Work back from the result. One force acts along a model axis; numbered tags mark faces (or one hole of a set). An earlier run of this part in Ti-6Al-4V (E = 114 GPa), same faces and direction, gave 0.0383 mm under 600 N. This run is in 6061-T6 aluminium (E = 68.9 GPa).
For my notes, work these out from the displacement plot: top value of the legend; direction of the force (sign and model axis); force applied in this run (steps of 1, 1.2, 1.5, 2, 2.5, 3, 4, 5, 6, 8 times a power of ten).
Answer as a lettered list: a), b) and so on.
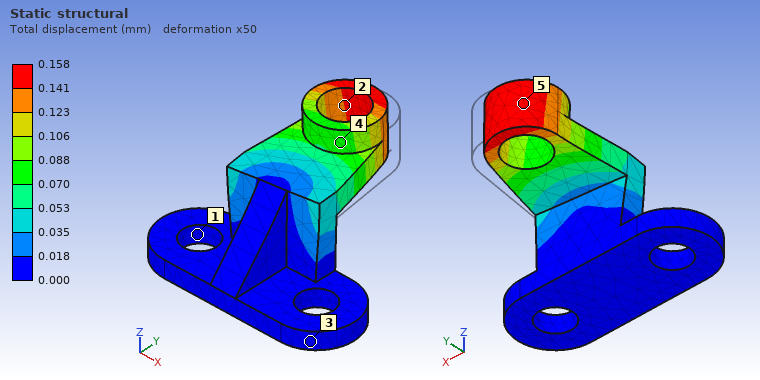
a) 0.158 mm
b) -X
c) 1.5 kN
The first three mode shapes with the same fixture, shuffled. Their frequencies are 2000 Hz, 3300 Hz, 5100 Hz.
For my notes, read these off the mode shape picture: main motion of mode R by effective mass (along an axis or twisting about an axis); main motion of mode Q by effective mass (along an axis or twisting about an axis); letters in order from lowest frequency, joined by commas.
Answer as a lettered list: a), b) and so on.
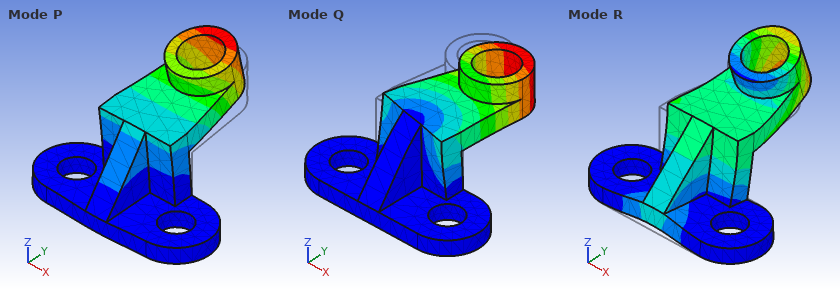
a) along Y
b) along X
c) P, Q, R
